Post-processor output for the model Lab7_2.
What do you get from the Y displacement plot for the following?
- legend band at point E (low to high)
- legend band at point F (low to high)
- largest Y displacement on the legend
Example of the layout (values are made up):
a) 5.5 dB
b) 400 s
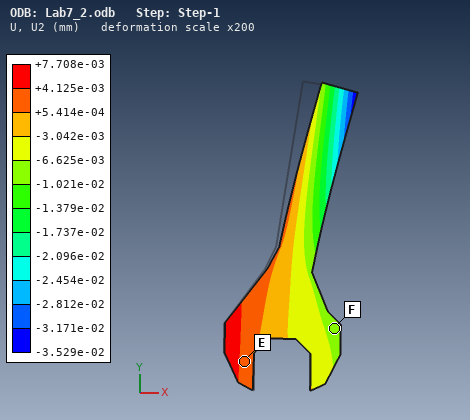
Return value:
a) +5.414e-04 to +4.125e-03 mm
b) -1.021e-02 to -6.625e-03 mm
c) +7.708e-03 mm
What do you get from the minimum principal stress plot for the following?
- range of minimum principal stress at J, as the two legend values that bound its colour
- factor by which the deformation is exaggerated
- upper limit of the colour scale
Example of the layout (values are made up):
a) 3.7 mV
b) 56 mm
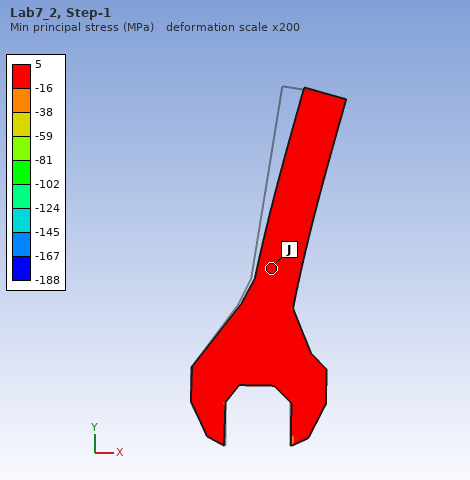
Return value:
a) -16 to 5 MPa
b) 200
c) 5 MPa
